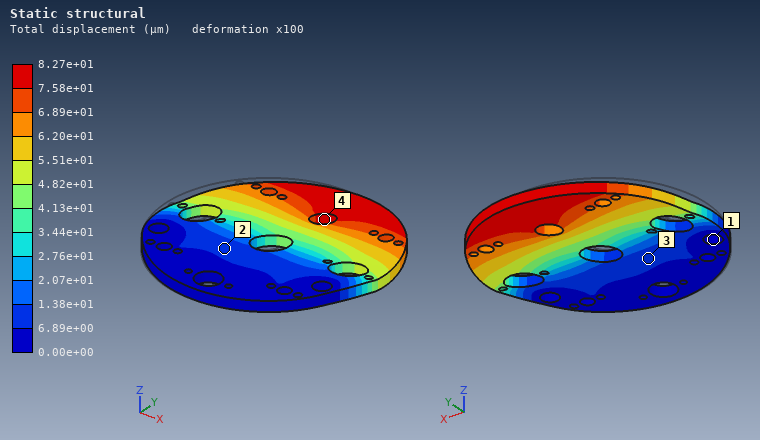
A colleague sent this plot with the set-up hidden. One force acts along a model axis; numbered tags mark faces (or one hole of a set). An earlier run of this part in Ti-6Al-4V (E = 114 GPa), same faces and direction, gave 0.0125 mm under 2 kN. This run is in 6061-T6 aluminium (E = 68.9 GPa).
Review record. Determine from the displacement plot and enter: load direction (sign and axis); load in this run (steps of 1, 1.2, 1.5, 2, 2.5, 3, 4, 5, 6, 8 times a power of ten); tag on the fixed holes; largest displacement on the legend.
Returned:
+X
8 kN
1
8.27e+01 µm
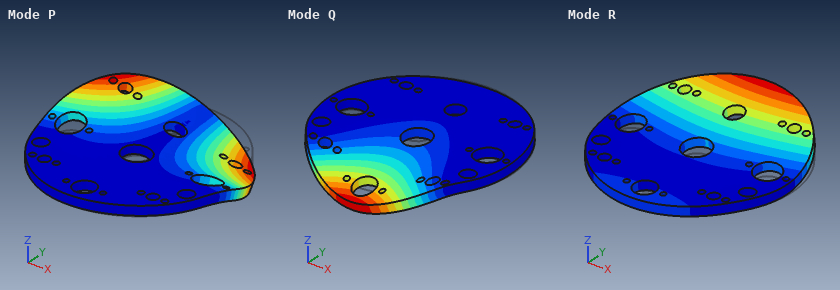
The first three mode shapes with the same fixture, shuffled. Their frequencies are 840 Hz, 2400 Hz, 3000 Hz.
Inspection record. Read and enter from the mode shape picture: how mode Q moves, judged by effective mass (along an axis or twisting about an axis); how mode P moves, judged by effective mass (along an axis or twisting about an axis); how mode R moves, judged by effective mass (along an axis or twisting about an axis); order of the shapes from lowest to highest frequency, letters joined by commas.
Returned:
along Z
twisting about Y
along Z
R, P, Q
